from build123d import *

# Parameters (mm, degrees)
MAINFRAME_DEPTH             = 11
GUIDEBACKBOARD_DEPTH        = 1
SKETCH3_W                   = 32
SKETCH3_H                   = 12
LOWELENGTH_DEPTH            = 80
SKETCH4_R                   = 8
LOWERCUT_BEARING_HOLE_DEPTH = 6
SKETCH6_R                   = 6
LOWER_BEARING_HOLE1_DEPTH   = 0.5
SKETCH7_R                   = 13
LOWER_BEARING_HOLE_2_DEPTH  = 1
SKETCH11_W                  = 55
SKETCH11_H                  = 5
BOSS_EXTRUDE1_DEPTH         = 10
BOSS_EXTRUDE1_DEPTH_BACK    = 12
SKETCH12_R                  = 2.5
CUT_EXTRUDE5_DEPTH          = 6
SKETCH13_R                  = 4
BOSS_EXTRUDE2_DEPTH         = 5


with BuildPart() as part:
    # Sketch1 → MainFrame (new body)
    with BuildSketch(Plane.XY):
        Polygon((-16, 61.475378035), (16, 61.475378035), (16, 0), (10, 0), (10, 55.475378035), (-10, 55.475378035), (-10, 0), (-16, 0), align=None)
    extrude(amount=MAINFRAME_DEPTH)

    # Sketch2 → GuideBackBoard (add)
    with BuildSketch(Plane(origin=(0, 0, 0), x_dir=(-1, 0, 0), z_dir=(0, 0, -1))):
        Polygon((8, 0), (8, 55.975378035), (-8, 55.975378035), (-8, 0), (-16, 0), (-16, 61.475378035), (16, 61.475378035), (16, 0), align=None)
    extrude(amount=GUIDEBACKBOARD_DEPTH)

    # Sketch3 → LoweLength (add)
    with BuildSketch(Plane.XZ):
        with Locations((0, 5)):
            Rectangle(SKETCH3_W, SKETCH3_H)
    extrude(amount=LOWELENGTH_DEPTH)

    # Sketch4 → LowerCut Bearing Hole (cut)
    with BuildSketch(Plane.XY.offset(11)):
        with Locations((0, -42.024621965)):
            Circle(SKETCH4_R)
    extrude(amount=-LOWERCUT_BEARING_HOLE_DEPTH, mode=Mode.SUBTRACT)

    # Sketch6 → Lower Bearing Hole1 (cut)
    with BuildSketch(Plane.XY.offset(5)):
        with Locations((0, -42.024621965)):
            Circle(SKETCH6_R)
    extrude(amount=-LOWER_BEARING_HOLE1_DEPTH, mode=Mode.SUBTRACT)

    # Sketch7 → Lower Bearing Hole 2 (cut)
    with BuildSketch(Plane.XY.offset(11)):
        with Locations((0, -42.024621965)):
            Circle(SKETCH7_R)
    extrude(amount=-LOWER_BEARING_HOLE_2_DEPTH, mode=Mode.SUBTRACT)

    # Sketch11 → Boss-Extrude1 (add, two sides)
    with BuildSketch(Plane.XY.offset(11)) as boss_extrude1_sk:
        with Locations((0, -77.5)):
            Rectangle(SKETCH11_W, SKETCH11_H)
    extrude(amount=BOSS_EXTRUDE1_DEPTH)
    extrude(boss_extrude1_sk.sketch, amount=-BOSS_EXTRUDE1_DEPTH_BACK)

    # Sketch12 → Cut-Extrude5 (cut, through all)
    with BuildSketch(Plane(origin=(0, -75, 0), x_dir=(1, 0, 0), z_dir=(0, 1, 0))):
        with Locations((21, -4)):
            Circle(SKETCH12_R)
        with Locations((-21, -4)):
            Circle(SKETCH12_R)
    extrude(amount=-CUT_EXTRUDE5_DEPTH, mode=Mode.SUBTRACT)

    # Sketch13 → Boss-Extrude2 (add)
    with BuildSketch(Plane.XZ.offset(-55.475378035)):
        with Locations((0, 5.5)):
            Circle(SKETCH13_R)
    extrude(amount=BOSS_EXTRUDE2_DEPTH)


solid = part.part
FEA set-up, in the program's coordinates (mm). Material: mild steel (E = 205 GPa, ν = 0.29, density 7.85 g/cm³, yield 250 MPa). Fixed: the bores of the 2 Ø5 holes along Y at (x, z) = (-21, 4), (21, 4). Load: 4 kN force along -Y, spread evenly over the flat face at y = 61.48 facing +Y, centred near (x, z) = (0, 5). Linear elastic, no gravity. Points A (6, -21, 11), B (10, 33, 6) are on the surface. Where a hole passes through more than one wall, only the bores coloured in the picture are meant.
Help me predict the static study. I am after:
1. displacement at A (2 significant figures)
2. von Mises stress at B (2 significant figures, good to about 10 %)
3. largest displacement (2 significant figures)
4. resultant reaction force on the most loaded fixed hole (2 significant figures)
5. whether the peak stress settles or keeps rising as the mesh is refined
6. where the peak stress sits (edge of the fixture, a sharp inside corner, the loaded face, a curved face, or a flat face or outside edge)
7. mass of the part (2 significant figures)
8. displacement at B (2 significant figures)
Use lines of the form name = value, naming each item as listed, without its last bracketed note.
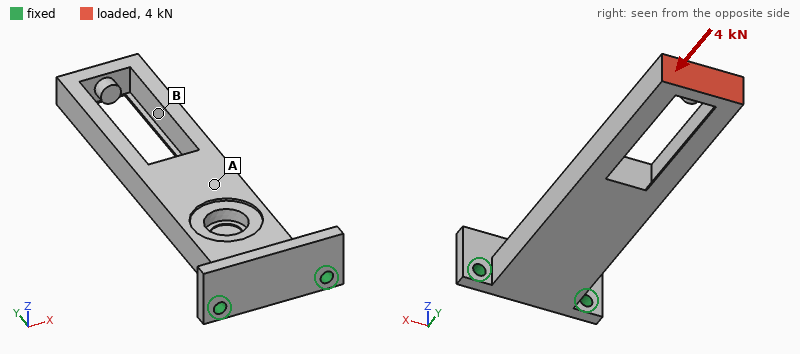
displacement at A = 12 µm
von Mises stress at B = 43 MPa
largest displacement = 44 µm
resultant reaction force on the most loaded fixed hole = 2.2 kN
whether the peak stress settles or keeps rising as the mesh is refined = keeps rising
where the peak stress sits = edge of the fixture
mass of the part = 340 g
displacement at B = 28 µm
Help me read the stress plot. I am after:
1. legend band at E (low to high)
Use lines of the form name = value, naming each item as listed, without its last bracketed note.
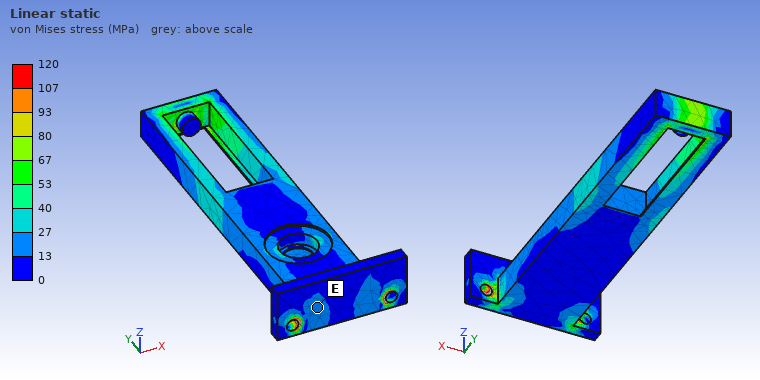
legend band at E = 13 to 27 MPa
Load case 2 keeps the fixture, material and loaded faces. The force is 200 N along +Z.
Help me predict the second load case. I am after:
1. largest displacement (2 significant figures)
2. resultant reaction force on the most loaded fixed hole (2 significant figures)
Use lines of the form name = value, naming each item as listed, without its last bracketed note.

largest displacement = 0.48 mm
resultant reaction force on the most loaded fixed hole = 190 N
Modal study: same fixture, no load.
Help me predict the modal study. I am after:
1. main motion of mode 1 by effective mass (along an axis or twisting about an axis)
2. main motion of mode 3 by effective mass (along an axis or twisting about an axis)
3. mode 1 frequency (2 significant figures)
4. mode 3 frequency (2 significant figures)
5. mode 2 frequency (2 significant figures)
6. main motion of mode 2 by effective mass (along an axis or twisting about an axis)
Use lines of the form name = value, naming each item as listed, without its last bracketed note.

main motion of mode 1 by effective mass = along Z
main motion of mode 3 by effective mass = along Z
mode 1 frequency = 410 Hz
mode 3 frequency = 2200 Hz
mode 2 frequency = 1100 Hz
main motion of mode 2 by effective mass = along X
